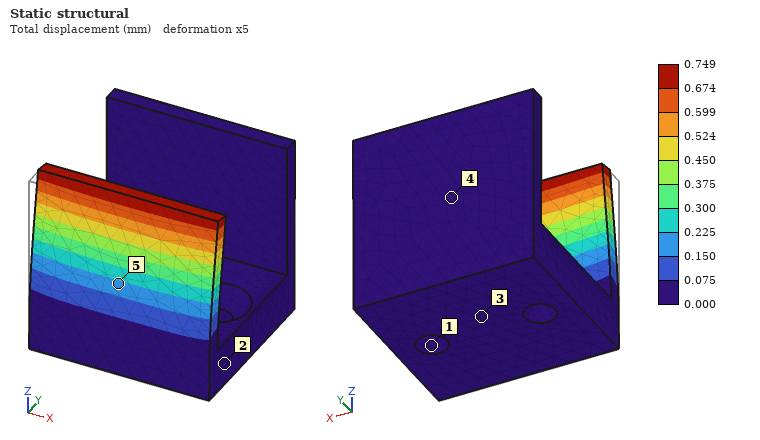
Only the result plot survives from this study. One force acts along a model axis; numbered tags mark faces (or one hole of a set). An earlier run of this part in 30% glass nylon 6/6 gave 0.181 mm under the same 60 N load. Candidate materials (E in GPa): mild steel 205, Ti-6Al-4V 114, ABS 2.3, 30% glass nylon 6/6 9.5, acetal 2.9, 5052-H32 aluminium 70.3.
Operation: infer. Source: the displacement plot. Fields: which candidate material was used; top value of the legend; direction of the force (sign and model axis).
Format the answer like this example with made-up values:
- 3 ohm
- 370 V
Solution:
- ABS
- 0.749 mm
- +Y
